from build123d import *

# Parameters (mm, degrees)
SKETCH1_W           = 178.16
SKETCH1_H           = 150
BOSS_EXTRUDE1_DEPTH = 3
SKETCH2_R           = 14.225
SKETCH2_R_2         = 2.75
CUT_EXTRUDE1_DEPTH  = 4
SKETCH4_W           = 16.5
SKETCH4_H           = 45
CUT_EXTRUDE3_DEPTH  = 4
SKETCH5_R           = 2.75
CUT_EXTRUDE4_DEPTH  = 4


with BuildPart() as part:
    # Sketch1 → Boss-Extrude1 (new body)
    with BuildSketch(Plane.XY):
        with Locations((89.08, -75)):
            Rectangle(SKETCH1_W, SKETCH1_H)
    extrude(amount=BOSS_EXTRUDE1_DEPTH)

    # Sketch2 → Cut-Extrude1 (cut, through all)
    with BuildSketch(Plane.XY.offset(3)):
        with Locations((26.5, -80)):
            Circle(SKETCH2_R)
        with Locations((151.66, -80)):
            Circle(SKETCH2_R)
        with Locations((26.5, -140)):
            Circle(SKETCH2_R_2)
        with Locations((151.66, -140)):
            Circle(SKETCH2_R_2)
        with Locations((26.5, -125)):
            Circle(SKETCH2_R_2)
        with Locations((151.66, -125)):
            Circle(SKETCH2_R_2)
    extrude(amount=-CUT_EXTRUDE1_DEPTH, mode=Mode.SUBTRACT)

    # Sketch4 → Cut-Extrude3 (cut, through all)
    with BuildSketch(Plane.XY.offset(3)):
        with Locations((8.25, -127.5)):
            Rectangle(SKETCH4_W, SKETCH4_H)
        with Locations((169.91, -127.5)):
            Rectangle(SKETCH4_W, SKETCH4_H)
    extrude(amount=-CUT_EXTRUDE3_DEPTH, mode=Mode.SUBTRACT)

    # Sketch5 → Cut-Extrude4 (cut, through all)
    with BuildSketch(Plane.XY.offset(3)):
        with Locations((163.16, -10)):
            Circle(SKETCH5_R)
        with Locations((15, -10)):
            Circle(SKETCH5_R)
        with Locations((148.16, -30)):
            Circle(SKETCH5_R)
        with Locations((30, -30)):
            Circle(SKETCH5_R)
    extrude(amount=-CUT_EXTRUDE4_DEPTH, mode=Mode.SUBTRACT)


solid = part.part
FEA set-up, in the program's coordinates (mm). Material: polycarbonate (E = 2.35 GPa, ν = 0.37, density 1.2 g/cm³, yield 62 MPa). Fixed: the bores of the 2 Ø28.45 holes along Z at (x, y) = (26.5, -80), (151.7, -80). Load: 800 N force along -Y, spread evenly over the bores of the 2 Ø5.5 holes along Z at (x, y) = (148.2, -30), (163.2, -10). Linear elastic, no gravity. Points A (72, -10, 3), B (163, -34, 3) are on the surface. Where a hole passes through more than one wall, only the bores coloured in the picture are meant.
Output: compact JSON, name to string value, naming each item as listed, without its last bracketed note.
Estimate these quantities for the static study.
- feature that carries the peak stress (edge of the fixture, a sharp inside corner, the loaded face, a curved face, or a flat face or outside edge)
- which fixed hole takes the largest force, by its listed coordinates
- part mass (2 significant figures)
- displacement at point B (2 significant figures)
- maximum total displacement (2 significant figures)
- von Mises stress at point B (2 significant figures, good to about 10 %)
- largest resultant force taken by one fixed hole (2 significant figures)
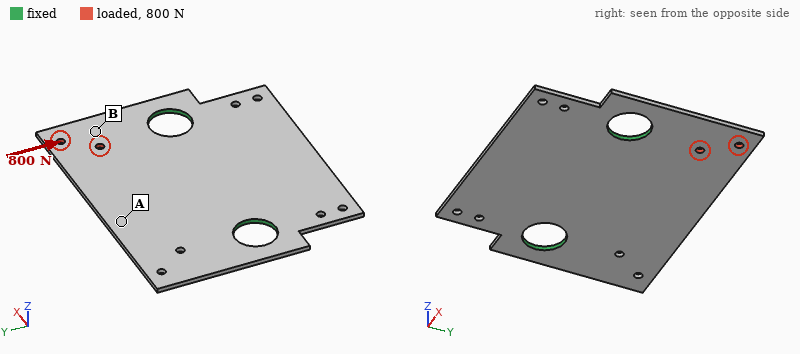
{"feature that carries the peak stress": "the loaded face", "which fixed hole takes the largest force, by its listed coordinates": "(151.7, -80)", "part mass": "86 g", "displacement at point B": "0.100 mm", "maximum total displacement": "0.18 mm", "von Mises stress at point B": "5.3 MPa", "largest resultant force taken by one fixed hole": "800 N"}
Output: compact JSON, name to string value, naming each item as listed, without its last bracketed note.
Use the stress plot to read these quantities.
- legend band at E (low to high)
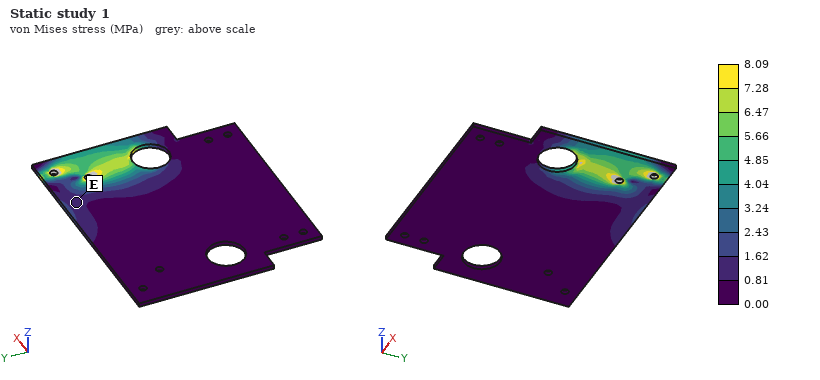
{"legend band at E": "0.81 to 1.62 MPa"}
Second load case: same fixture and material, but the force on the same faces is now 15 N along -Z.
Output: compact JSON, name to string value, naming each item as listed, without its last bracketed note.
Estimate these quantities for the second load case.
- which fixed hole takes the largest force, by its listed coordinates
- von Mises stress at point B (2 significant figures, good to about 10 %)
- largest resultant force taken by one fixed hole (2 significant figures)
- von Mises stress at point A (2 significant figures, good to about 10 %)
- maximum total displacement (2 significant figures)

{"which fixed hole takes the largest force, by its listed coordinates": "(151.7, -80)", "von Mises stress at point B": "1.6 MPa", "largest resultant force taken by one fixed hole": "15 N", "von Mises stress at point A": "0.92 MPa", "maximum total displacement": "2.3 mm"}
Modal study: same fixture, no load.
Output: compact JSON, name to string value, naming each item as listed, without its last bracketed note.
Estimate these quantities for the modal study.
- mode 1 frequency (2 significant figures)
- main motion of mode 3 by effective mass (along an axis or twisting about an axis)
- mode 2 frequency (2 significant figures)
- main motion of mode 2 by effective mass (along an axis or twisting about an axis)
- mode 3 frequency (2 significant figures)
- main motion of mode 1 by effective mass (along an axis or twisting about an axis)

{"mode 1 frequency": "130 Hz", "main motion of mode 3 by effective mass": "twisting about Y", "mode 2 frequency": "170 Hz", "main motion of mode 2 by effective mass": "along Z", "mode 3 frequency": "200 Hz", "main motion of mode 1 by effective mass": "along Z"}
